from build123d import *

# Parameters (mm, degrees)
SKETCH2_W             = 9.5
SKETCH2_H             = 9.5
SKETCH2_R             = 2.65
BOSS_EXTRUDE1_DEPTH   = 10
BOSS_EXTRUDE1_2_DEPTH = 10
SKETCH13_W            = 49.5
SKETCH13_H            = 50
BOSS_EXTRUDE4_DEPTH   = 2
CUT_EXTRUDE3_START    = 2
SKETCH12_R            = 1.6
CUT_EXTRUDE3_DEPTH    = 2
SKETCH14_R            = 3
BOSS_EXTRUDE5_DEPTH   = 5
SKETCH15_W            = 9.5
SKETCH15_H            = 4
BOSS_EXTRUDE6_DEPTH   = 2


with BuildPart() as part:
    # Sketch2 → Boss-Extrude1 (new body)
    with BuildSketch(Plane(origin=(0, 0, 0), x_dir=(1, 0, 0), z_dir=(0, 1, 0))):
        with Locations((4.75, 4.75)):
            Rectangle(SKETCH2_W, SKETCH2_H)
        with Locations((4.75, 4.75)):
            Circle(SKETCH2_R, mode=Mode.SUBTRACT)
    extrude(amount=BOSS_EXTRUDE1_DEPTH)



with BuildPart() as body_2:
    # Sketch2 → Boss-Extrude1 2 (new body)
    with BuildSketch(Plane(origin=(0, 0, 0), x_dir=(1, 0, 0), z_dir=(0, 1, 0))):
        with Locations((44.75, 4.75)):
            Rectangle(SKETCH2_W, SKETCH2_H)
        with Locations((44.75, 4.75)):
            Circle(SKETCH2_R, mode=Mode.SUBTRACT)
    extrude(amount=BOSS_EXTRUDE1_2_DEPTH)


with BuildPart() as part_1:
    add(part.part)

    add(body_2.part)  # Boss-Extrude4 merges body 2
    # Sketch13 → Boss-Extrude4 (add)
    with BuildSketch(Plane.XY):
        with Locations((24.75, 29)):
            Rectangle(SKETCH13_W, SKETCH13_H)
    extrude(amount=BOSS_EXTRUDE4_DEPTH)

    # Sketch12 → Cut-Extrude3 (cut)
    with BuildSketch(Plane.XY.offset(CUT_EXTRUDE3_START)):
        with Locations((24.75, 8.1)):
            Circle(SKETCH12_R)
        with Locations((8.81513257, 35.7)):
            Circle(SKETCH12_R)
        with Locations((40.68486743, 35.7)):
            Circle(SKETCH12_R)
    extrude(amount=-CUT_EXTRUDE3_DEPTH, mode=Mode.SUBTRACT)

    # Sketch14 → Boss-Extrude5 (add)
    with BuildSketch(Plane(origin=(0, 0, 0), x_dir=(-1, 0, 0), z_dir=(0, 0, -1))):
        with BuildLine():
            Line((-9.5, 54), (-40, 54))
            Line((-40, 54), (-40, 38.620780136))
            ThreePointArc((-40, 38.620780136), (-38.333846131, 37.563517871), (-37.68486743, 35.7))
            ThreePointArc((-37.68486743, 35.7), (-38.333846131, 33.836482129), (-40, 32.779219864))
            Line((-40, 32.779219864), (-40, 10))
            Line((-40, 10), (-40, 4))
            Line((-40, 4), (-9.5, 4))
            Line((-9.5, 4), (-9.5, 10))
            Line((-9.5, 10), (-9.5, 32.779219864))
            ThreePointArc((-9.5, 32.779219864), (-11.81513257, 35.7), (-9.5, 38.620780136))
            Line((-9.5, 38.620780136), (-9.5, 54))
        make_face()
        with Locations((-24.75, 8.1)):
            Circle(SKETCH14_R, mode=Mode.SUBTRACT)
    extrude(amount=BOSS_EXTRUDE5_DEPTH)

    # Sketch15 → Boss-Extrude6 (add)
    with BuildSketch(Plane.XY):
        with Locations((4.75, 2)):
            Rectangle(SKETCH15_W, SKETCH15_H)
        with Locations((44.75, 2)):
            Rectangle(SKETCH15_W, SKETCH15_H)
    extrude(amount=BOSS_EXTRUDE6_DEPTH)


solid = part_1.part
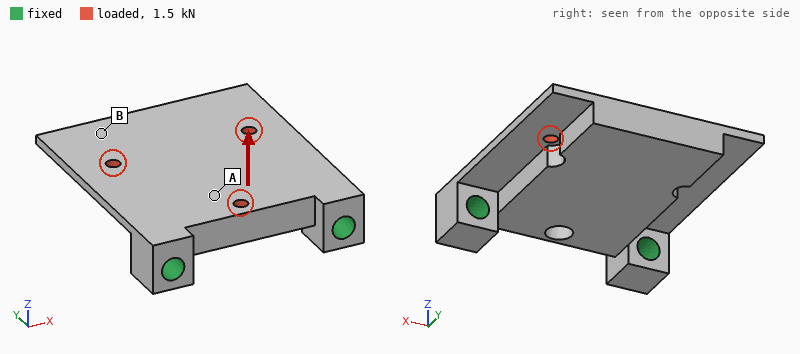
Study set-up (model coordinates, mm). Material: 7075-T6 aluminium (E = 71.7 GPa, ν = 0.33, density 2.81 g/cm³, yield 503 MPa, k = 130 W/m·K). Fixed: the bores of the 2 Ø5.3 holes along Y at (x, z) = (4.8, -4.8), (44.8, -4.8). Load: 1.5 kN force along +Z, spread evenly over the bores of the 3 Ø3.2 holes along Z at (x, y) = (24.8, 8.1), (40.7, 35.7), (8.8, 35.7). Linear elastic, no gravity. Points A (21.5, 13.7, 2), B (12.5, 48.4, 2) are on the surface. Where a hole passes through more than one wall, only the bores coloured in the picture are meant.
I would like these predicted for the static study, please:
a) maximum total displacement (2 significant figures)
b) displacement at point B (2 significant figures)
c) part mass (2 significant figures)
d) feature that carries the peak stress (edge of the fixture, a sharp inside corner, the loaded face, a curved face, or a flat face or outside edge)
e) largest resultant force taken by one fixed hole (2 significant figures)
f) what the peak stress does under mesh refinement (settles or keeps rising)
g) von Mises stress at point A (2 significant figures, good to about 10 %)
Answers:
0.46 mm
0.40 mm
39 g
a sharp inside corner
870 N
keeps rising
57 MPa
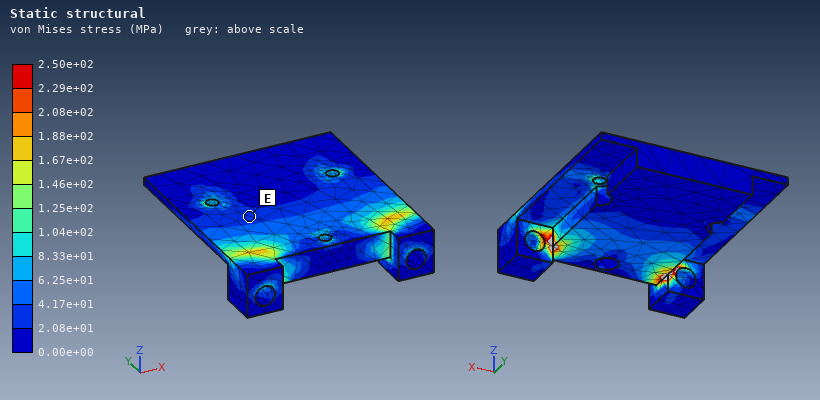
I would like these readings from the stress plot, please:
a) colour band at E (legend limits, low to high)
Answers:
2.08e+01 to 4.17e+01 MPa
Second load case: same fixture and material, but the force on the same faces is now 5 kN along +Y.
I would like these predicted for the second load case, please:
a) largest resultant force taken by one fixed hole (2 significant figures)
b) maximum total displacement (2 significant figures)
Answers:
2.6 kN
0.17 mm
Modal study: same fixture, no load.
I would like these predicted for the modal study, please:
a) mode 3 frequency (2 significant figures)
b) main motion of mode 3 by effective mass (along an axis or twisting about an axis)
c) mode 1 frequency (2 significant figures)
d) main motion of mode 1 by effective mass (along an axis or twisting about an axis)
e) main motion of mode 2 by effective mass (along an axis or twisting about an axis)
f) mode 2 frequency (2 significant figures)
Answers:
8900 Hz
along X
1800 Hz
along Z
twisting about Y
5400 Hz
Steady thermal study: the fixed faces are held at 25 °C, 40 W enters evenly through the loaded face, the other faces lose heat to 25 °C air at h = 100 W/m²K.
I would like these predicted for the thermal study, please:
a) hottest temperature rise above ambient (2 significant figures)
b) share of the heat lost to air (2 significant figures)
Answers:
39 K
32 %
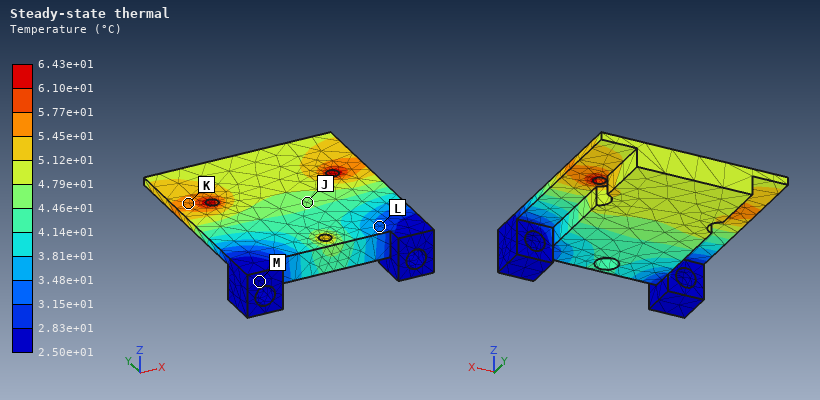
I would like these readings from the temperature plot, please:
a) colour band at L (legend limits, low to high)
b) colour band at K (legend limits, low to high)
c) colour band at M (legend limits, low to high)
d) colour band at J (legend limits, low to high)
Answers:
3.15e+01 to 3.48e+01 °C
5.45e+01 to 5.77e+01 °C
2.50e+01 to 2.83e+01 °C
4.46e+01 to 4.79e+01 °C
